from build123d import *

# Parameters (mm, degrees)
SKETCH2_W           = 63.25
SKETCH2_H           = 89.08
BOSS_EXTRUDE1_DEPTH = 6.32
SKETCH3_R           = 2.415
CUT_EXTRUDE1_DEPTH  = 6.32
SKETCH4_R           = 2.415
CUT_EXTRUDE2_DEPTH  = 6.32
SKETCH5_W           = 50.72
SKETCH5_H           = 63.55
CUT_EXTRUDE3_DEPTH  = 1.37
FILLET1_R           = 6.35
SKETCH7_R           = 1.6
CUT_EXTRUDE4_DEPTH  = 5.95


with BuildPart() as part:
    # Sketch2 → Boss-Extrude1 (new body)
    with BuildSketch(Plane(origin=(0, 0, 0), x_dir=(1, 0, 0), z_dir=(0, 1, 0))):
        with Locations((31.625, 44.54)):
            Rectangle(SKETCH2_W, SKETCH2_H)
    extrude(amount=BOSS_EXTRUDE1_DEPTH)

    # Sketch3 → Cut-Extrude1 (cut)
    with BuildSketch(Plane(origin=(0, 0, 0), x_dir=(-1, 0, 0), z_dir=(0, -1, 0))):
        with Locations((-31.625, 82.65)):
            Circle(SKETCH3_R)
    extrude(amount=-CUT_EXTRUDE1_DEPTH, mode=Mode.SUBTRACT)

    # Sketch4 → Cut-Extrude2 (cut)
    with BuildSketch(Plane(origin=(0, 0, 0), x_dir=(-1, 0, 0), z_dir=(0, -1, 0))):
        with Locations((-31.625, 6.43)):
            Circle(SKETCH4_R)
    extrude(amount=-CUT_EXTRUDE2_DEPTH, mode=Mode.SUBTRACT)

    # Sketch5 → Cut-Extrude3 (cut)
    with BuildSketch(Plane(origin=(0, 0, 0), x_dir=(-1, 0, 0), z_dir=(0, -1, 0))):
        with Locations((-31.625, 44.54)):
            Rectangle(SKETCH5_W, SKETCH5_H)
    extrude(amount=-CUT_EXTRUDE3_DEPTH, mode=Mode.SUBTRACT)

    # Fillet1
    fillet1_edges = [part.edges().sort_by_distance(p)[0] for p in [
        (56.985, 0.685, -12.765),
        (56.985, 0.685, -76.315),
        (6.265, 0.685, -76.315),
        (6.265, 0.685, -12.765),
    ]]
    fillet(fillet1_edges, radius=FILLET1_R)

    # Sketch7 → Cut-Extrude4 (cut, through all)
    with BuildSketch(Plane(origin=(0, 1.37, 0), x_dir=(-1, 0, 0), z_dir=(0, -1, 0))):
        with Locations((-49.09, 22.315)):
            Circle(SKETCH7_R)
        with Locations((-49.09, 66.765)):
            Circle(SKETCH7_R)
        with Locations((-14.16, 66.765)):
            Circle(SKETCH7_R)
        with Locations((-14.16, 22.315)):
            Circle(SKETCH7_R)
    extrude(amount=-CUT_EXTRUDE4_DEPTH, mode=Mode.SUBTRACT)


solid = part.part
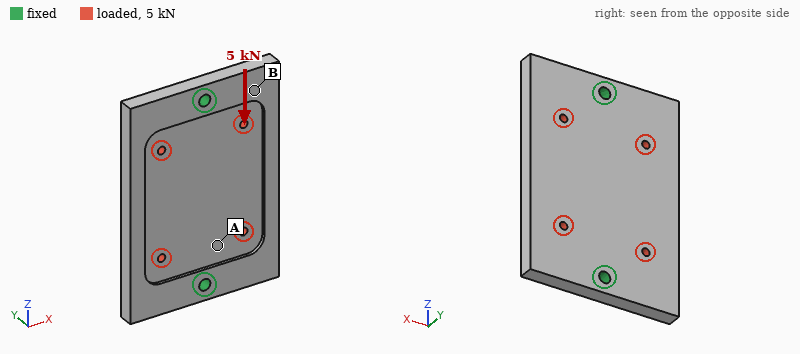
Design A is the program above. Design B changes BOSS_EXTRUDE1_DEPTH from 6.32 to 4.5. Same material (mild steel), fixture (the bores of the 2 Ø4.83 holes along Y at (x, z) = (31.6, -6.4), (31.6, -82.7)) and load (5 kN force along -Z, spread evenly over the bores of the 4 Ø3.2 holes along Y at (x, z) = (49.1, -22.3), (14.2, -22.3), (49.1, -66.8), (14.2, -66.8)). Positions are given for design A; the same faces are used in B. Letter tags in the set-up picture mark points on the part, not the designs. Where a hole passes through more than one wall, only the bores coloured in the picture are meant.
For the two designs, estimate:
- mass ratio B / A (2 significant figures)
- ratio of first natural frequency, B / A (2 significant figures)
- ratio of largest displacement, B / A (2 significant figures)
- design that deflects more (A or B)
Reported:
0.67
0.74
1.6
B
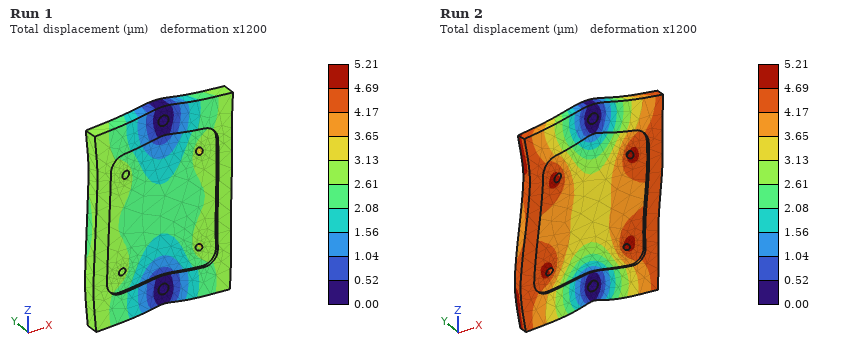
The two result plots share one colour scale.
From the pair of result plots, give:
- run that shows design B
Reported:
Run 2
